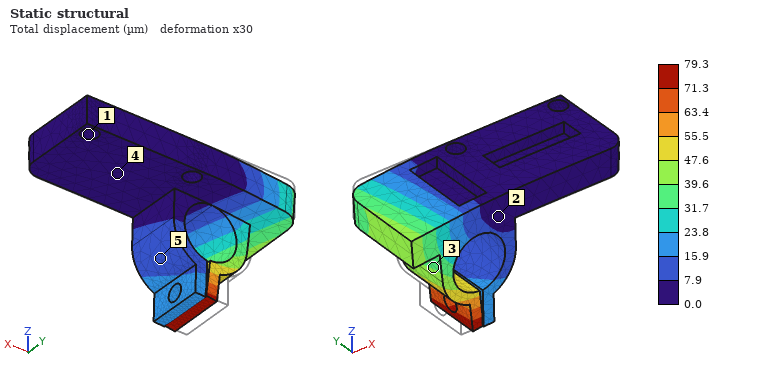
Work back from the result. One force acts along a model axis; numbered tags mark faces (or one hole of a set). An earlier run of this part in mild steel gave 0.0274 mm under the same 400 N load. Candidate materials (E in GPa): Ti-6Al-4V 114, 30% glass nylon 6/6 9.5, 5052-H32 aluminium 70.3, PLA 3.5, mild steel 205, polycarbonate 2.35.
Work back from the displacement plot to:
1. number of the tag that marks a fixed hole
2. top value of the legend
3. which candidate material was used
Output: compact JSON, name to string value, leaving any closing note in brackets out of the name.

{"number of the tag that marks a fixed hole": "1", "top value of the legend": "79.3 µm", "which candidate material was used": "5052-H32 aluminium"}
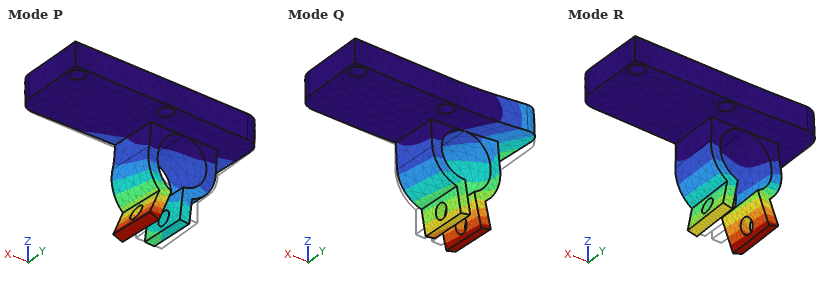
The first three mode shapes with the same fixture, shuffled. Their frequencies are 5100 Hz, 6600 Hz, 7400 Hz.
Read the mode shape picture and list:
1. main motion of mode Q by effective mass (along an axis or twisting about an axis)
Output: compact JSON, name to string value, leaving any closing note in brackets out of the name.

{"main motion of mode Q by effective mass": "along Z"}
